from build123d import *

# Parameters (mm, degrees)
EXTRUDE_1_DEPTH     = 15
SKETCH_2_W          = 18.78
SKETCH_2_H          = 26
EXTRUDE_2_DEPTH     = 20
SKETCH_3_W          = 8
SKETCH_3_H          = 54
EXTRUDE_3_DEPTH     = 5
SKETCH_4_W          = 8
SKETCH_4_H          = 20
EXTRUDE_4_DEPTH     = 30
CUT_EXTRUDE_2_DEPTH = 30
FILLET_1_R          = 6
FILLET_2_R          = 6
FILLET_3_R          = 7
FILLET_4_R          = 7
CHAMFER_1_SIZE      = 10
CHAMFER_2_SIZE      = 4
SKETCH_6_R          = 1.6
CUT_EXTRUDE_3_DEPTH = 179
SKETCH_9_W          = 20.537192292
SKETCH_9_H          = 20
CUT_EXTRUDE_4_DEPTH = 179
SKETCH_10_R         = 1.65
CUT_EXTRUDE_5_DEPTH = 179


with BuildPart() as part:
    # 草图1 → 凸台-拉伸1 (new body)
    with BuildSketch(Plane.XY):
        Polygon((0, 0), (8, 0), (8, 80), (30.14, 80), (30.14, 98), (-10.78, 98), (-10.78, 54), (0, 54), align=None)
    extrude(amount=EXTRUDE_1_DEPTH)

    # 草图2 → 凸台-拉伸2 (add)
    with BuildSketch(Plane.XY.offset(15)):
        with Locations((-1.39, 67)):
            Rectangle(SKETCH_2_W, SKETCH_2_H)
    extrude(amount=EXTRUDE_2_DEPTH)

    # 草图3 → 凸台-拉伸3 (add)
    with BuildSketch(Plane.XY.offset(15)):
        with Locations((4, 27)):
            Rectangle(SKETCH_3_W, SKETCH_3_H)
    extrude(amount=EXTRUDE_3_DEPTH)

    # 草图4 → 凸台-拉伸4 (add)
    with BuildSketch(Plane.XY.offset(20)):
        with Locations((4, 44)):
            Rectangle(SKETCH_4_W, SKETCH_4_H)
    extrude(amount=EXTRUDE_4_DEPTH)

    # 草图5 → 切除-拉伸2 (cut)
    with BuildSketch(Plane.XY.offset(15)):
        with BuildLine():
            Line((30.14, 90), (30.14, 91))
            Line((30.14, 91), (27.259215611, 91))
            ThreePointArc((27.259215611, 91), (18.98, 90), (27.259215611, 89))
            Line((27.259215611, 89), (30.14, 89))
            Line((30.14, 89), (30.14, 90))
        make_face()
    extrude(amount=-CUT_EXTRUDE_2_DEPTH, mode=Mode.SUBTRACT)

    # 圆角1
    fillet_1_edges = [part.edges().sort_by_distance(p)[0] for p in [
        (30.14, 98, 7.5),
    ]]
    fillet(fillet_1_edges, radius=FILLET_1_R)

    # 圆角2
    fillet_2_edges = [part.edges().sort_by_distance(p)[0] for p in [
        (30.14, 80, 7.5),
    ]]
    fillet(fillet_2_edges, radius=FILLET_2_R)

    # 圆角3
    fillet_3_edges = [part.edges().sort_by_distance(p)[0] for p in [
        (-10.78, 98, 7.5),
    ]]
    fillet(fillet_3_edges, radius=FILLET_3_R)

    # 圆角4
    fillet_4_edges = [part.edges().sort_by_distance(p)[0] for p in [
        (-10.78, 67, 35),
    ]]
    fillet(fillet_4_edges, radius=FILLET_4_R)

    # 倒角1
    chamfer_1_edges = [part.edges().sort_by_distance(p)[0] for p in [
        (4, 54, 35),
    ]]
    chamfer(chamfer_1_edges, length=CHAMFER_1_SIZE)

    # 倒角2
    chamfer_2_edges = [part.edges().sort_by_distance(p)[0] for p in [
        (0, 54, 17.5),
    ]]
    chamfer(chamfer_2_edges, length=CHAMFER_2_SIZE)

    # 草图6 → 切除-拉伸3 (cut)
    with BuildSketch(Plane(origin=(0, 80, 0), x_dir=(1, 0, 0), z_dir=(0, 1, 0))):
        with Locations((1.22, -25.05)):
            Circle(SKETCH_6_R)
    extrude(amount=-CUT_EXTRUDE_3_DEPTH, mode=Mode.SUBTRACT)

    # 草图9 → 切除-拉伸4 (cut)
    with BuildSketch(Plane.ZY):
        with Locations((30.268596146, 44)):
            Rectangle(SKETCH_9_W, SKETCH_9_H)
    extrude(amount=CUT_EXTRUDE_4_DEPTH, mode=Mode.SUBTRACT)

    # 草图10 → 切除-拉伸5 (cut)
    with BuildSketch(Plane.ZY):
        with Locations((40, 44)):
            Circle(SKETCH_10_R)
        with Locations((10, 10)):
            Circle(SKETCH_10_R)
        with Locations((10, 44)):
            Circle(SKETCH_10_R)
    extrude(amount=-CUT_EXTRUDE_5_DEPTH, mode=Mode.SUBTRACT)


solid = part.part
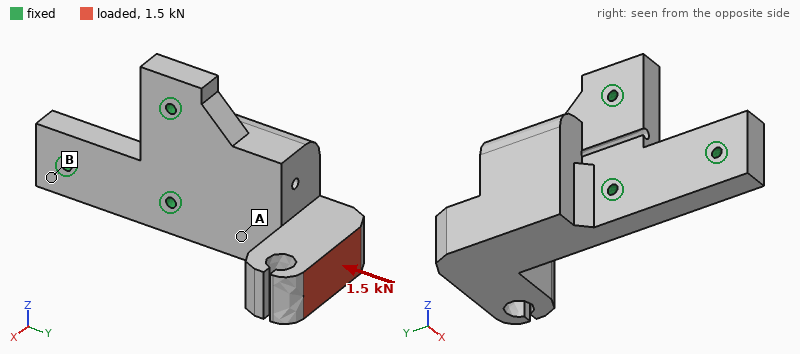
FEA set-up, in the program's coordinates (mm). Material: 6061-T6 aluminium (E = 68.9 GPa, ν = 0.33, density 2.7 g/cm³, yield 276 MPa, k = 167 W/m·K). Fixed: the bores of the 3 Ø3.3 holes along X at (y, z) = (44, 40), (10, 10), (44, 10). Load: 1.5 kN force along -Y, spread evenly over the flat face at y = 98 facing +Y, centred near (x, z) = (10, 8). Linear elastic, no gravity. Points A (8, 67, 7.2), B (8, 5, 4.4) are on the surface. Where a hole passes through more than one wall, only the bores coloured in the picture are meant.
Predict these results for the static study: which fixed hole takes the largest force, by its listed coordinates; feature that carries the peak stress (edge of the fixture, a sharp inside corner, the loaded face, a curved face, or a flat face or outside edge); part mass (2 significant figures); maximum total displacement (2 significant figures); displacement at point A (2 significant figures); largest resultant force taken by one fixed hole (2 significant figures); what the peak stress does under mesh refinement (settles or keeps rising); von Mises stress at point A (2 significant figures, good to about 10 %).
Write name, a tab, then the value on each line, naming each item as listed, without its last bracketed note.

which fixed hole takes the largest force, by its listed coordinates	(44, 10)
feature that carries the peak stress	edge of the fixture
part mass	110 g
maximum total displacement	93 µm
displacement at point A	23 µm
largest resultant force taken by one fixed hole	1.4 kN
what the peak stress does under mesh refinement	keeps rising
von Mises stress at point A	18 MPa
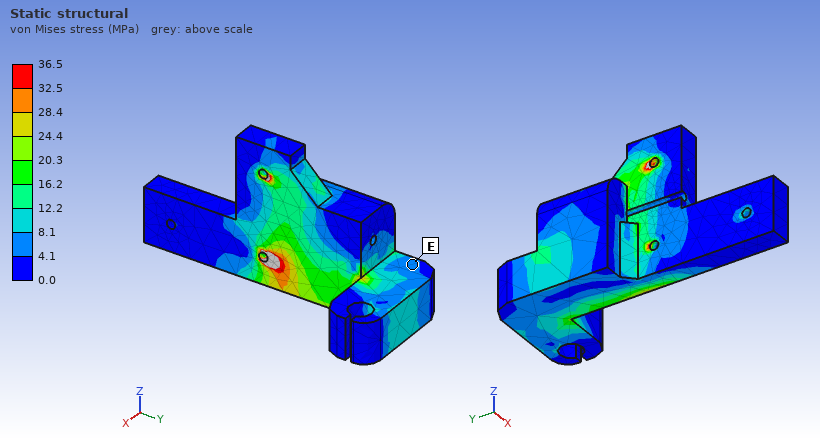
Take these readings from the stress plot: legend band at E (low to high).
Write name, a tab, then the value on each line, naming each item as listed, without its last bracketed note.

legend band at E	4.1 to 8.1 MPa
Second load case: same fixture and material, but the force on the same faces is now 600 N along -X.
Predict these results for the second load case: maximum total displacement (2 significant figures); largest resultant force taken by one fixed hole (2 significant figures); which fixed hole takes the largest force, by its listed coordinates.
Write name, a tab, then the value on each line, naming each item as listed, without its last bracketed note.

maximum total displacement	0.22 mm
largest resultant force taken by one fixed hole	790 N
which fixed hole takes the largest force, by its listed coordinates	(44, 10)
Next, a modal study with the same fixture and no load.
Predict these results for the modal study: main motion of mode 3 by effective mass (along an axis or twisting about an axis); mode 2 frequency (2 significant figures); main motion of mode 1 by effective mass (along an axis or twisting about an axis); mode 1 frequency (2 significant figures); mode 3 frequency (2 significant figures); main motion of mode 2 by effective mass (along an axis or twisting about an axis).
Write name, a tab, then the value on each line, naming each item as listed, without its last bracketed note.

main motion of mode 3 by effective mass	along Z
mode 2 frequency	5100 Hz
main motion of mode 1 by effective mass	along X
mode 1 frequency	1700 Hz
mode 3 frequency	7700 Hz
main motion of mode 2 by effective mass	along Z
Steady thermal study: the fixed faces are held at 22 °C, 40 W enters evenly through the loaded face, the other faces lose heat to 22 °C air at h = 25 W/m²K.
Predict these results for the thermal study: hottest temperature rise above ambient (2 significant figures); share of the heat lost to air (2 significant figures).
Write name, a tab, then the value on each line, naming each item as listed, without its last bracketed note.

hottest temperature rise above ambient	40 K
share of the heat lost to air	9.2 %
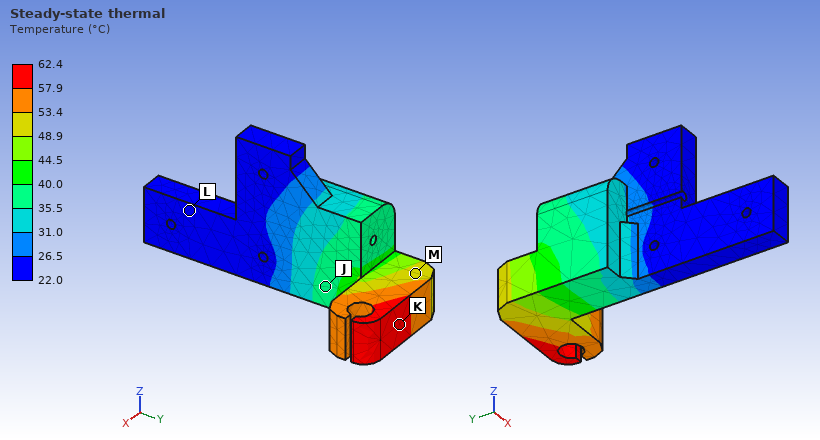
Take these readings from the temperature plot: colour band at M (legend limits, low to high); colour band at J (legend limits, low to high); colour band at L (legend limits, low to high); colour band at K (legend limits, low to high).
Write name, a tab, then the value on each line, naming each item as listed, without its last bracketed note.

colour band at M	48.9 to 53.4 °C
colour band at J	35.5 to 40.0 °C
colour band at L	22.0 to 26.5 °C
colour band at K	57.9 to 62.4 °C
